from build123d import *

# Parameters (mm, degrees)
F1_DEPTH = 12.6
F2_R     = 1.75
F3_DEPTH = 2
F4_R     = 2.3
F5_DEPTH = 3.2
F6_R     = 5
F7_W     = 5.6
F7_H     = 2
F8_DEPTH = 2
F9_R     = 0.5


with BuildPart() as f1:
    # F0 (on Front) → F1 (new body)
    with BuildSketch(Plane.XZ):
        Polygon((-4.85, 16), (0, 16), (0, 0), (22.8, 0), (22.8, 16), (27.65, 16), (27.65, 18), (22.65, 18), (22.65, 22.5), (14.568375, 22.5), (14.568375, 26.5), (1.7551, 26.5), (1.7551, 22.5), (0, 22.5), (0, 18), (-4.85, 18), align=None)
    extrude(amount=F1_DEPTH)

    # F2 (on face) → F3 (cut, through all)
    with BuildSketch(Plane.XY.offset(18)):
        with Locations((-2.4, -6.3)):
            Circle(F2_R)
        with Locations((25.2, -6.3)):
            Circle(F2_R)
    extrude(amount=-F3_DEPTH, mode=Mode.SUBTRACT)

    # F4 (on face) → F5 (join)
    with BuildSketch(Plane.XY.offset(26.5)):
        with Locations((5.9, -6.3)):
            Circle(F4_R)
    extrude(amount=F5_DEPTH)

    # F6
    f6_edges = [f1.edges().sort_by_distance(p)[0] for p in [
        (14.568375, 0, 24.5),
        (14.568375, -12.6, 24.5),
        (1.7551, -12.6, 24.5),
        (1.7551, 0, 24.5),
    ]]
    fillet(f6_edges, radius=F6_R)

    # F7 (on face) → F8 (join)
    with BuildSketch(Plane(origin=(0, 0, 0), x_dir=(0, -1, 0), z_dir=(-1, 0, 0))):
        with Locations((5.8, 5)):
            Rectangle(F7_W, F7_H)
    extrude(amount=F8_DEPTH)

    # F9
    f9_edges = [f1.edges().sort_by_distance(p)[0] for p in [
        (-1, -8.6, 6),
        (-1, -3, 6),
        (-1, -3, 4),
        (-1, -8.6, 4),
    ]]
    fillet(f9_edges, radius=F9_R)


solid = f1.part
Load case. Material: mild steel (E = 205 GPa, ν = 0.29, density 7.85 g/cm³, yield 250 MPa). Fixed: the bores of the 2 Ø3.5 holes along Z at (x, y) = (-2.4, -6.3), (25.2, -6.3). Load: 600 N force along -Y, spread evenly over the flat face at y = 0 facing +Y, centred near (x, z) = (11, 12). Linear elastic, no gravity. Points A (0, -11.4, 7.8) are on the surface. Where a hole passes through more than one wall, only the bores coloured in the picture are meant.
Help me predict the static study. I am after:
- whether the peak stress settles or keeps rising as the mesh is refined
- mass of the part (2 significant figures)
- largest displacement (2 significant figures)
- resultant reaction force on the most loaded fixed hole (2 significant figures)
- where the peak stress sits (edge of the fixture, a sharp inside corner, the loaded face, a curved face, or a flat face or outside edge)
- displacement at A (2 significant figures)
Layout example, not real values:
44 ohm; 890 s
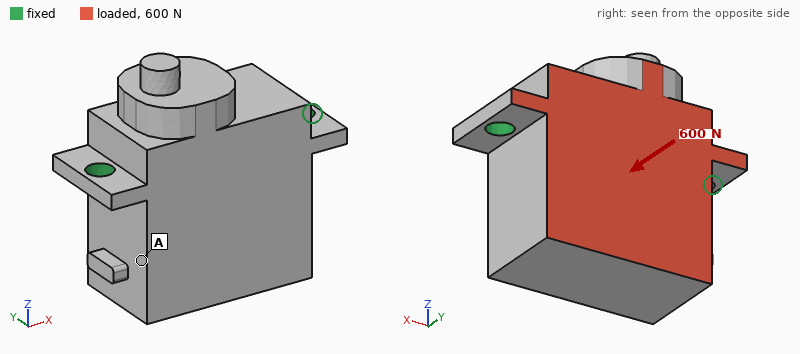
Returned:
keeps rising; 57 g; 16 µm; 300 N; edge of the fixture; 9.7 µm
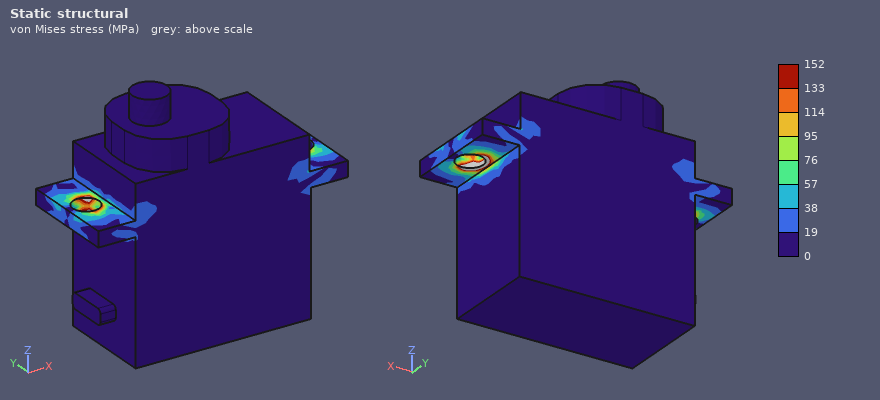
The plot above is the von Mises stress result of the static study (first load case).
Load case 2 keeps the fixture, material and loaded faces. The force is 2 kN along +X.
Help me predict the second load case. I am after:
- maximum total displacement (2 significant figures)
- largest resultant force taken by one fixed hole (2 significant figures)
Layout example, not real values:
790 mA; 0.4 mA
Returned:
4.8 µm; 1.2 kN
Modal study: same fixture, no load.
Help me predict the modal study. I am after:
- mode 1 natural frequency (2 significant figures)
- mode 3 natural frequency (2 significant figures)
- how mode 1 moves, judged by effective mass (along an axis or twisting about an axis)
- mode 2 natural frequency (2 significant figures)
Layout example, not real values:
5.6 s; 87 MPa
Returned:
4400 Hz; 18 kHz; along Y; 18 kHz
